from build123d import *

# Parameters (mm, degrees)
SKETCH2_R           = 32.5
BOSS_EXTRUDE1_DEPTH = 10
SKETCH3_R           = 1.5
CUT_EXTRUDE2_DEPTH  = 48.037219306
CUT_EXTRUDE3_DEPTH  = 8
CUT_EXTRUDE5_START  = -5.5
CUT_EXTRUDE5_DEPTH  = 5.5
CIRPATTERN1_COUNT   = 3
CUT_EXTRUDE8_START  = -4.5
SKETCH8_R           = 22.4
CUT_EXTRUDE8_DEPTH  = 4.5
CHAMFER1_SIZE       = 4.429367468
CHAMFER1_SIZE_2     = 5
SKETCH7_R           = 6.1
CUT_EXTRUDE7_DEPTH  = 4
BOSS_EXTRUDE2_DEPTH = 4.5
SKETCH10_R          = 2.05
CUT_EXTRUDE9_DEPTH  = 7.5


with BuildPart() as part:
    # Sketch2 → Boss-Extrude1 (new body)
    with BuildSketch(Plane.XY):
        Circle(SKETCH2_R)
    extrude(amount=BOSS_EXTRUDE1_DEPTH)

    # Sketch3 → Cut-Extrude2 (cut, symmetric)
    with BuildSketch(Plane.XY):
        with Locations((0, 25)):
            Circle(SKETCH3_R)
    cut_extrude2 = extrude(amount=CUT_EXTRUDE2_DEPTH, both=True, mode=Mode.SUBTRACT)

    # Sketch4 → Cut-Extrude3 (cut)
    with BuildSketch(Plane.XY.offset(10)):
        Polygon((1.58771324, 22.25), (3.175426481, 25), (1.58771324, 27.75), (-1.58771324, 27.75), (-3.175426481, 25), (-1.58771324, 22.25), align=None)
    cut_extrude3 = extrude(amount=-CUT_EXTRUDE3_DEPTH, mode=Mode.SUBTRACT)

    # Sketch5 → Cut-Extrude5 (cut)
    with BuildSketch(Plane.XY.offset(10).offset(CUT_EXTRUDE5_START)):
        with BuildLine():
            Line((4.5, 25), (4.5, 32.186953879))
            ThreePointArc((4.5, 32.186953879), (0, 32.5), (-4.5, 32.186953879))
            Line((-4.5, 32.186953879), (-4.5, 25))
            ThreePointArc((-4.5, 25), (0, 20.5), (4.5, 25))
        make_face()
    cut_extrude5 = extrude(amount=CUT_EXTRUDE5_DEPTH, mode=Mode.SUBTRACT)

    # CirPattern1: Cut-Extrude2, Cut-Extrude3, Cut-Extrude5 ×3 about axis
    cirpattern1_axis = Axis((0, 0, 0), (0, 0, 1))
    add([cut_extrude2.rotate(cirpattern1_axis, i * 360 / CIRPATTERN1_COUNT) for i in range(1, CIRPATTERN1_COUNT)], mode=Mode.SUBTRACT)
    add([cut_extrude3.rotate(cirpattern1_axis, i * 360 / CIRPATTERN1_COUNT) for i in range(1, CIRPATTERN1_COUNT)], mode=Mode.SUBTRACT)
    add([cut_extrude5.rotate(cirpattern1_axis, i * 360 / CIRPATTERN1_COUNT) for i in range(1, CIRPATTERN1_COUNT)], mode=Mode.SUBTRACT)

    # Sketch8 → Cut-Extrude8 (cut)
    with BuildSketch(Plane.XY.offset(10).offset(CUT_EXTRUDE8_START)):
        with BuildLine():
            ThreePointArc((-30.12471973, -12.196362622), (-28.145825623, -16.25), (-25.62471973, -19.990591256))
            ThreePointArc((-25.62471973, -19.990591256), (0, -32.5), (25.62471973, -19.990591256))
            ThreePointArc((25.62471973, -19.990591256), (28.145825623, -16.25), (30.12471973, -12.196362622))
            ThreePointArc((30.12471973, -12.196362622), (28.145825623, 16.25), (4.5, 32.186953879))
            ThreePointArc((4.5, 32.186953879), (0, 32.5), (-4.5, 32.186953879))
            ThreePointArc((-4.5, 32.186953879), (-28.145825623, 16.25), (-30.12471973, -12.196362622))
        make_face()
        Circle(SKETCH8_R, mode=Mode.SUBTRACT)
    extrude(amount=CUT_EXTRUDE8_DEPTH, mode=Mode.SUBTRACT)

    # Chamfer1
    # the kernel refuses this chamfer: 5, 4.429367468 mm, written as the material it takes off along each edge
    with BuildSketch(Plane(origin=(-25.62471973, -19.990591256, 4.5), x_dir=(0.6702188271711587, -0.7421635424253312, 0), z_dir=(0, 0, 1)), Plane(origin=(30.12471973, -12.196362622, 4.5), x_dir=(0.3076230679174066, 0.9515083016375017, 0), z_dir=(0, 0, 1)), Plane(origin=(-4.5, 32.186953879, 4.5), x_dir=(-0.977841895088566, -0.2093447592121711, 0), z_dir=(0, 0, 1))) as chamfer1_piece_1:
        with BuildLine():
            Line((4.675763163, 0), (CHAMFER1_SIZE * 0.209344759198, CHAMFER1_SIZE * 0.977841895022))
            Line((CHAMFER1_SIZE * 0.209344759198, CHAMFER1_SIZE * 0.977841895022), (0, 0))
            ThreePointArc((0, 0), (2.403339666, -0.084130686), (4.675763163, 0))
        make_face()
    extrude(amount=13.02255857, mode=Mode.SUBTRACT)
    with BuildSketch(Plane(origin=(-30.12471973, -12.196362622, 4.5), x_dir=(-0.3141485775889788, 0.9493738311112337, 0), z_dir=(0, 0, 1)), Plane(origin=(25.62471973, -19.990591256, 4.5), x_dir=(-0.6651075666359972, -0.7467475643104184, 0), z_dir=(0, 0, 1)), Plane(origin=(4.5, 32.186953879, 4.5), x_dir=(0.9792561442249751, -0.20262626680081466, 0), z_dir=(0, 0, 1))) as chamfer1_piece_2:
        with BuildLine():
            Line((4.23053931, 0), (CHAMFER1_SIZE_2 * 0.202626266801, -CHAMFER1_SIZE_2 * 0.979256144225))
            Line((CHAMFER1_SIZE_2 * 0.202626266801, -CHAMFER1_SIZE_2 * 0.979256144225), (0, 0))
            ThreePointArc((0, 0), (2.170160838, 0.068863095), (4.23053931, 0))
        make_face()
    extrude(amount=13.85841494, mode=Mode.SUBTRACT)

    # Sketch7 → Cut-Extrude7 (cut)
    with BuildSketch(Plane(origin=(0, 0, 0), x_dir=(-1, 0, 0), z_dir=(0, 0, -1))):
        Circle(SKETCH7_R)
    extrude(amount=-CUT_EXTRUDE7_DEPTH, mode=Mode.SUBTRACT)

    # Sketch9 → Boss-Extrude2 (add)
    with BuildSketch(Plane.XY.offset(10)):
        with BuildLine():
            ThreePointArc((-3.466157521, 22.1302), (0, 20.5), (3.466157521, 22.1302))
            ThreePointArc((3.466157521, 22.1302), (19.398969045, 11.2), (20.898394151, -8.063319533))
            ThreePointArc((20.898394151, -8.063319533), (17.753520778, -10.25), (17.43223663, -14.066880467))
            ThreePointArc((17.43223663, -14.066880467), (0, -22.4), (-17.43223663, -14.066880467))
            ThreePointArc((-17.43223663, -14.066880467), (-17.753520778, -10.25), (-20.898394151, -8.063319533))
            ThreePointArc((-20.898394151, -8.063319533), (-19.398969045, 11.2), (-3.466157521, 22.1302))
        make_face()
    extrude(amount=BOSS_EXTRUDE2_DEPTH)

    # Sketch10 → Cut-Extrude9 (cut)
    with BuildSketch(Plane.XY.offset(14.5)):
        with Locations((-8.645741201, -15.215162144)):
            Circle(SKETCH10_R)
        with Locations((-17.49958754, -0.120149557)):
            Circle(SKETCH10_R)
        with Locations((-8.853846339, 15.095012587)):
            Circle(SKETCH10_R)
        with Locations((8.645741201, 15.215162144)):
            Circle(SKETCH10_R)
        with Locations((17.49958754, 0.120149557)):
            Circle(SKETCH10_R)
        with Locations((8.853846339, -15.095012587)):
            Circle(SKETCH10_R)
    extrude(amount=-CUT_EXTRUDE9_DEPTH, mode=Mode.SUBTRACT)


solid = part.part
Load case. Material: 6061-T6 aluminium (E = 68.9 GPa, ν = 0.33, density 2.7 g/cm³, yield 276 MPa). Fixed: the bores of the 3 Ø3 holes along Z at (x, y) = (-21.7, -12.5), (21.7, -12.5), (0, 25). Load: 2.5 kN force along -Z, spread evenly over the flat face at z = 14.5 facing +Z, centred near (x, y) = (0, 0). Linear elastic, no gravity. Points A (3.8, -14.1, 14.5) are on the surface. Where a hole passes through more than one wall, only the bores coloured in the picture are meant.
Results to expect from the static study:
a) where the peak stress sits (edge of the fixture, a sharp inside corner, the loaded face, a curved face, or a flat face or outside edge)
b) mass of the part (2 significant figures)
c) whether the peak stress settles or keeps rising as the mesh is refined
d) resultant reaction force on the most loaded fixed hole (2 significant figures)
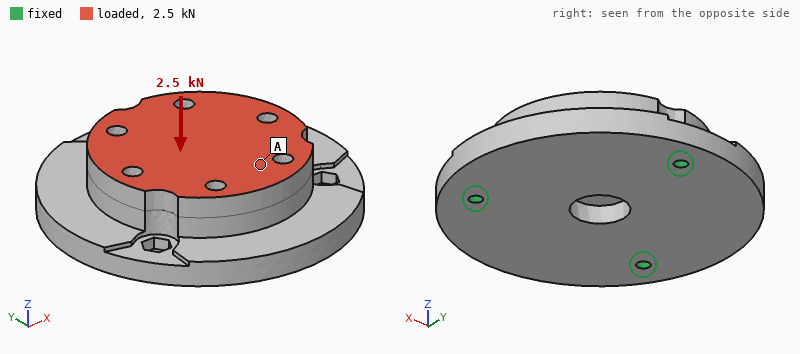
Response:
edge of the fixture
82 g
keeps rising
970 N
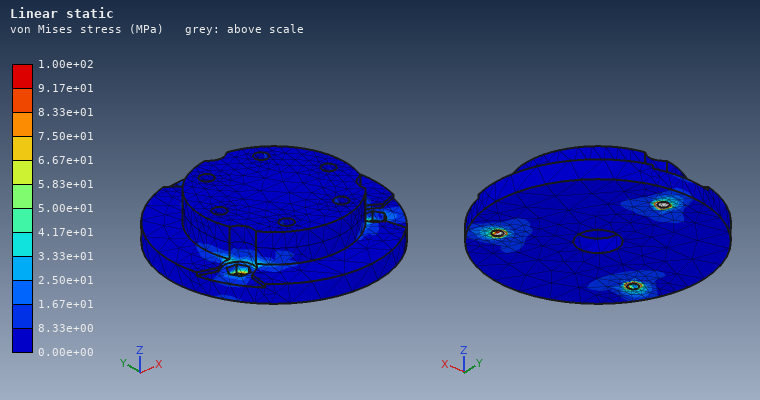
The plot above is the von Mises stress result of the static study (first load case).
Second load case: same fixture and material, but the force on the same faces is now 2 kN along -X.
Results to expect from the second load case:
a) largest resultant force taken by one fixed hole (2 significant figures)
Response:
1.0 kN
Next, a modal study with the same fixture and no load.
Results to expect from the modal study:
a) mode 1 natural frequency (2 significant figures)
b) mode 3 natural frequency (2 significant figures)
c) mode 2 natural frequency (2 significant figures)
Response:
9300 Hz
9300 Hz
9300 Hz
